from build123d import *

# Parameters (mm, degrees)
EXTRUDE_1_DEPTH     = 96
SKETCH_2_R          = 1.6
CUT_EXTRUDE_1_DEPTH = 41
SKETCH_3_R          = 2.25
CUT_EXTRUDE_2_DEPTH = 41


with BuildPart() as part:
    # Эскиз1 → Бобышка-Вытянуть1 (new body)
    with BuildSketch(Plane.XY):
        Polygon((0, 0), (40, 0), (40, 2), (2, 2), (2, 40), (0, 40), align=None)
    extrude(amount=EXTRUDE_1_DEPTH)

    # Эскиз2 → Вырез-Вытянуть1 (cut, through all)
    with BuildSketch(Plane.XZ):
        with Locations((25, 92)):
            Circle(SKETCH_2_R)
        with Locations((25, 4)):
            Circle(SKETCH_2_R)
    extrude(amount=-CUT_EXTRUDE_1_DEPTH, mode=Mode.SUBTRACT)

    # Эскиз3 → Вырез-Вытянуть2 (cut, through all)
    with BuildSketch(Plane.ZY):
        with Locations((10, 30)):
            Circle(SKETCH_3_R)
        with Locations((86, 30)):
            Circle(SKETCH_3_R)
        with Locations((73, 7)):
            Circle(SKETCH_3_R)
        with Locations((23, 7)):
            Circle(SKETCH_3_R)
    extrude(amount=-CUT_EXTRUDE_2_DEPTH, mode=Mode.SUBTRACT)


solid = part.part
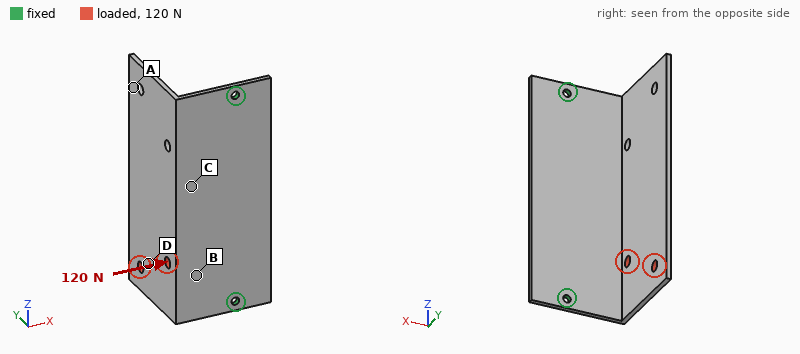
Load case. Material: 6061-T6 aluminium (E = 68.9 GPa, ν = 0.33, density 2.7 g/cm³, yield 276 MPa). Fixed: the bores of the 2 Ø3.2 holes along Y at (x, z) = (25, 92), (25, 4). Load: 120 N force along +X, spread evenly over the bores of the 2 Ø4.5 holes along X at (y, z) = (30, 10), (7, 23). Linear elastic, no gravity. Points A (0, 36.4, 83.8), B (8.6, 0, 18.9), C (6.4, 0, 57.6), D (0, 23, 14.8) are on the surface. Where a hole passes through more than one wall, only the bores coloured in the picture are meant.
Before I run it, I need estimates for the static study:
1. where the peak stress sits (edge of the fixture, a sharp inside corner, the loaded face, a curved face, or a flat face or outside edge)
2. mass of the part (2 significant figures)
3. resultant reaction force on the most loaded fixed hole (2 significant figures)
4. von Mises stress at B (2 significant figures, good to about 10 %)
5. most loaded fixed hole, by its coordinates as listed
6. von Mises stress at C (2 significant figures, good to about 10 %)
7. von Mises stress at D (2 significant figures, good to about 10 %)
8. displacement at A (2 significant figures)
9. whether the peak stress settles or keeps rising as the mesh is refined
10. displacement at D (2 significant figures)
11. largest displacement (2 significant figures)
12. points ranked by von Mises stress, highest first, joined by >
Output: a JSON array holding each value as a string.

["edge of the fixture", "40 g", "100 N", "45 MPa", "(25, 4)", "22 MPa", "29 MPa", "0.53 mm", "keeps rising", "0.67 mm", "1.2 mm", "B > D > C > A"]
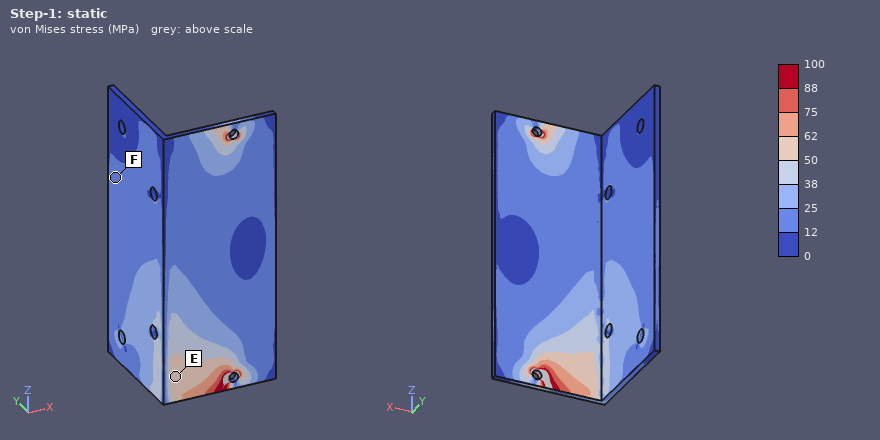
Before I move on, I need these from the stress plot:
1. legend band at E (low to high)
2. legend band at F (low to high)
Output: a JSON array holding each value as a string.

["50 to 62 MPa", "12 to 25 MPa"]
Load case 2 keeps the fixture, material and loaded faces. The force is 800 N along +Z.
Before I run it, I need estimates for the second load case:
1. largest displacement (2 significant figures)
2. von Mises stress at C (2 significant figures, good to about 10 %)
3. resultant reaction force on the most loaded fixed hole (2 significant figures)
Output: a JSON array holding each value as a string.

["0.82 mm", "32 MPa", "490 N"]
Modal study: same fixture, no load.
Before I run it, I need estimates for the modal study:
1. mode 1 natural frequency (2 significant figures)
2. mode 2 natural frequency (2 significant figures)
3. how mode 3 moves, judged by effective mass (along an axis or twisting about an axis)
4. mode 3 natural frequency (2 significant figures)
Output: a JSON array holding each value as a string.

["430 Hz", "910 Hz", "along Y", "1100 Hz"]
